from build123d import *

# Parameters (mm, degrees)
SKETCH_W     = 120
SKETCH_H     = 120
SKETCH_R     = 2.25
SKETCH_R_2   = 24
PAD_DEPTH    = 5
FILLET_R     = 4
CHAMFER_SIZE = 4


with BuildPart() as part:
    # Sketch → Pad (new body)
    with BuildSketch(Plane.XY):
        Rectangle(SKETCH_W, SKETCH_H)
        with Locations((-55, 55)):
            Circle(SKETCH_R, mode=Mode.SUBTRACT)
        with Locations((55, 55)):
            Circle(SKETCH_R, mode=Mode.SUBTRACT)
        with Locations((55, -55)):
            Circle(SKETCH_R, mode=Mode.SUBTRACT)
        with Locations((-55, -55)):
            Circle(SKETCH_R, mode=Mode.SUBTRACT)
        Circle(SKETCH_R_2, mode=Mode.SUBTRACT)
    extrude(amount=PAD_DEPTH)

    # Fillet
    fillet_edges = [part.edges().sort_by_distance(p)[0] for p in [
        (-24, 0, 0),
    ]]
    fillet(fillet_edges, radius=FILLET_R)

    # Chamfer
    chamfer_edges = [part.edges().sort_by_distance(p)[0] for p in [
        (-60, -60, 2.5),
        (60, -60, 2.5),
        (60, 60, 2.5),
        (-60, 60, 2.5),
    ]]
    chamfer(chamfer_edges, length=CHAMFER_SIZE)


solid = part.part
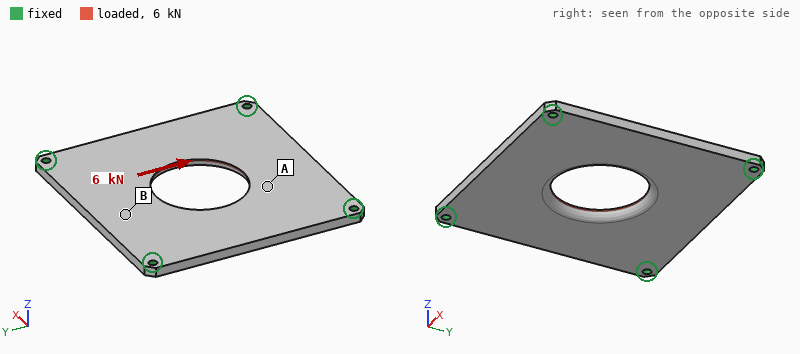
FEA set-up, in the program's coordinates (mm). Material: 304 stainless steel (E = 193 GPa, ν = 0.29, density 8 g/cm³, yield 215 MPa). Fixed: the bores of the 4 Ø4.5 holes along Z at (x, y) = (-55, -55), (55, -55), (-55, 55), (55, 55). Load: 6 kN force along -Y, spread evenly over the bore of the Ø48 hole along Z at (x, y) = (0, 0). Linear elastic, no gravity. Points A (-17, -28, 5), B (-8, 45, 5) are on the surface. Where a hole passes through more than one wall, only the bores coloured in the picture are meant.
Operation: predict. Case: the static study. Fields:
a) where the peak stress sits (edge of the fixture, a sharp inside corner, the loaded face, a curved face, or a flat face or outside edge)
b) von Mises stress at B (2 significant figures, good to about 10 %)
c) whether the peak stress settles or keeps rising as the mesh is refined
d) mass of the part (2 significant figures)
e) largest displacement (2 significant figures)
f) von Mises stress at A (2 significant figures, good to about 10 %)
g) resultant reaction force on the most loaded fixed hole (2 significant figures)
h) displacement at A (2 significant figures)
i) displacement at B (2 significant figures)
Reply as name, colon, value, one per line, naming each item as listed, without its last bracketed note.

where the peak stress sits: edge of the fixture
von Mises stress at B: 6.8 MPa
whether the peak stress settles or keeps rising as the mesh is refined: keeps rising
mass of the part: 500 g
largest displacement: 11 µm
von Mises stress at A: 17 MPa
resultant reaction force on the most loaded fixed hole: 1.7 kN
displacement at A: 7.0 µm
displacement at B: 9.3 µm
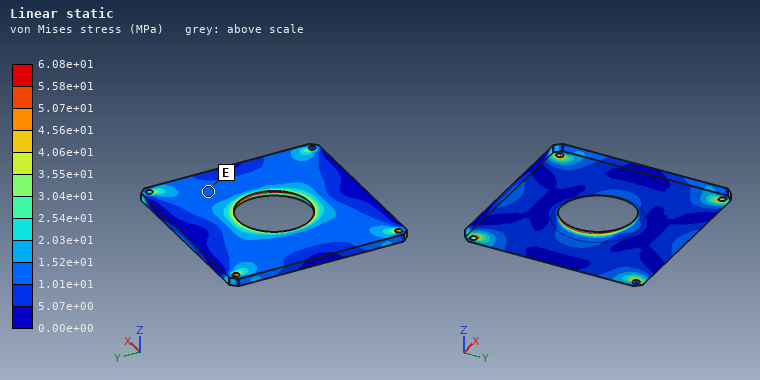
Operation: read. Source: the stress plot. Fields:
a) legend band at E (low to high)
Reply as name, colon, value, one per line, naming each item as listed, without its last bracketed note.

legend band at E: 1.01e+01 to 1.52e+01 MPa
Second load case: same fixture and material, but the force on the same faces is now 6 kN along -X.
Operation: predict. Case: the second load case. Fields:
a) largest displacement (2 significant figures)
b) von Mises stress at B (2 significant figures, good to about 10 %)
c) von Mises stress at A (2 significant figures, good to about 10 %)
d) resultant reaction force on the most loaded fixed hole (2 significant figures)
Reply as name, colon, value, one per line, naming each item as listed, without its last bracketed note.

largest displacement: 11 µm
von Mises stress at B: 11 MPa
von Mises stress at A: 14 MPa
resultant reaction force on the most loaded fixed hole: 1.7 kN
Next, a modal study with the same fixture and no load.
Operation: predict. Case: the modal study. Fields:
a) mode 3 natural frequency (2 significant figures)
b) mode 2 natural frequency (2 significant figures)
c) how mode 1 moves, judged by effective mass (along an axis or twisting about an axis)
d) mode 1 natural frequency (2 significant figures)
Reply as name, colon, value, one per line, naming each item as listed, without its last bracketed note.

mode 3 natural frequency: 2100 Hz
mode 2 natural frequency: 2100 Hz
how mode 1 moves, judged by effective mass: along Z
mode 1 natural frequency: 1300 Hz
